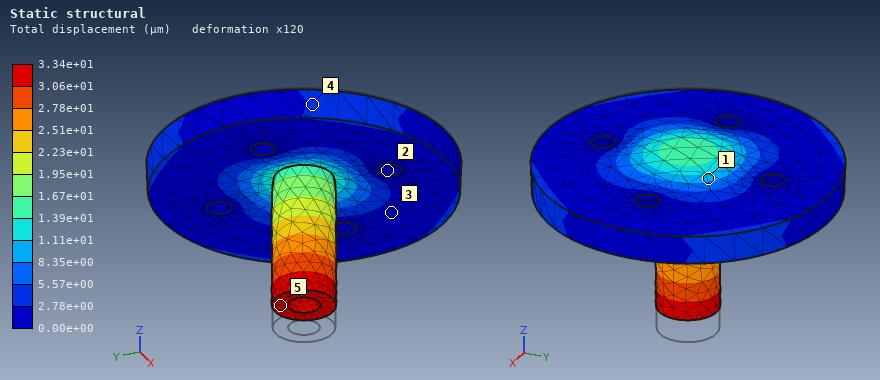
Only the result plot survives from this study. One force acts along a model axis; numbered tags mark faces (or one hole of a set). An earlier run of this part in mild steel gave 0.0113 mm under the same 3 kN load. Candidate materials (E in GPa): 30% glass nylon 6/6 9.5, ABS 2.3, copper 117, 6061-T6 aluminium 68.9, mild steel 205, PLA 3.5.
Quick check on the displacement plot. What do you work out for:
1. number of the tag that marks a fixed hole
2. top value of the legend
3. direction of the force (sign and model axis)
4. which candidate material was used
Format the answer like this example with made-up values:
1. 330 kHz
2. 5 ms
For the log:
1. 2
2. 3.34e+01 µm
3. +Z
4. 6061-T6 aluminium
